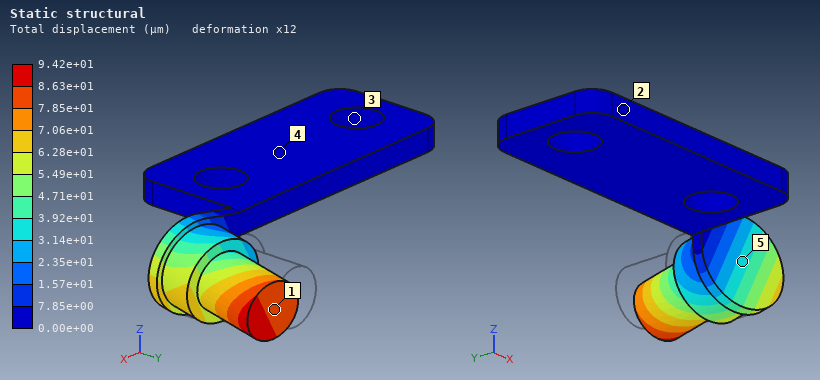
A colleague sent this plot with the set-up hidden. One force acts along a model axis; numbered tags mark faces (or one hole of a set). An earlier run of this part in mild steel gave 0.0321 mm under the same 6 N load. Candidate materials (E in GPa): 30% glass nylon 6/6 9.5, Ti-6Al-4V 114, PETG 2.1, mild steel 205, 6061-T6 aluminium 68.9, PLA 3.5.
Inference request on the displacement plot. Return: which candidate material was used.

6061-T6 aluminium
